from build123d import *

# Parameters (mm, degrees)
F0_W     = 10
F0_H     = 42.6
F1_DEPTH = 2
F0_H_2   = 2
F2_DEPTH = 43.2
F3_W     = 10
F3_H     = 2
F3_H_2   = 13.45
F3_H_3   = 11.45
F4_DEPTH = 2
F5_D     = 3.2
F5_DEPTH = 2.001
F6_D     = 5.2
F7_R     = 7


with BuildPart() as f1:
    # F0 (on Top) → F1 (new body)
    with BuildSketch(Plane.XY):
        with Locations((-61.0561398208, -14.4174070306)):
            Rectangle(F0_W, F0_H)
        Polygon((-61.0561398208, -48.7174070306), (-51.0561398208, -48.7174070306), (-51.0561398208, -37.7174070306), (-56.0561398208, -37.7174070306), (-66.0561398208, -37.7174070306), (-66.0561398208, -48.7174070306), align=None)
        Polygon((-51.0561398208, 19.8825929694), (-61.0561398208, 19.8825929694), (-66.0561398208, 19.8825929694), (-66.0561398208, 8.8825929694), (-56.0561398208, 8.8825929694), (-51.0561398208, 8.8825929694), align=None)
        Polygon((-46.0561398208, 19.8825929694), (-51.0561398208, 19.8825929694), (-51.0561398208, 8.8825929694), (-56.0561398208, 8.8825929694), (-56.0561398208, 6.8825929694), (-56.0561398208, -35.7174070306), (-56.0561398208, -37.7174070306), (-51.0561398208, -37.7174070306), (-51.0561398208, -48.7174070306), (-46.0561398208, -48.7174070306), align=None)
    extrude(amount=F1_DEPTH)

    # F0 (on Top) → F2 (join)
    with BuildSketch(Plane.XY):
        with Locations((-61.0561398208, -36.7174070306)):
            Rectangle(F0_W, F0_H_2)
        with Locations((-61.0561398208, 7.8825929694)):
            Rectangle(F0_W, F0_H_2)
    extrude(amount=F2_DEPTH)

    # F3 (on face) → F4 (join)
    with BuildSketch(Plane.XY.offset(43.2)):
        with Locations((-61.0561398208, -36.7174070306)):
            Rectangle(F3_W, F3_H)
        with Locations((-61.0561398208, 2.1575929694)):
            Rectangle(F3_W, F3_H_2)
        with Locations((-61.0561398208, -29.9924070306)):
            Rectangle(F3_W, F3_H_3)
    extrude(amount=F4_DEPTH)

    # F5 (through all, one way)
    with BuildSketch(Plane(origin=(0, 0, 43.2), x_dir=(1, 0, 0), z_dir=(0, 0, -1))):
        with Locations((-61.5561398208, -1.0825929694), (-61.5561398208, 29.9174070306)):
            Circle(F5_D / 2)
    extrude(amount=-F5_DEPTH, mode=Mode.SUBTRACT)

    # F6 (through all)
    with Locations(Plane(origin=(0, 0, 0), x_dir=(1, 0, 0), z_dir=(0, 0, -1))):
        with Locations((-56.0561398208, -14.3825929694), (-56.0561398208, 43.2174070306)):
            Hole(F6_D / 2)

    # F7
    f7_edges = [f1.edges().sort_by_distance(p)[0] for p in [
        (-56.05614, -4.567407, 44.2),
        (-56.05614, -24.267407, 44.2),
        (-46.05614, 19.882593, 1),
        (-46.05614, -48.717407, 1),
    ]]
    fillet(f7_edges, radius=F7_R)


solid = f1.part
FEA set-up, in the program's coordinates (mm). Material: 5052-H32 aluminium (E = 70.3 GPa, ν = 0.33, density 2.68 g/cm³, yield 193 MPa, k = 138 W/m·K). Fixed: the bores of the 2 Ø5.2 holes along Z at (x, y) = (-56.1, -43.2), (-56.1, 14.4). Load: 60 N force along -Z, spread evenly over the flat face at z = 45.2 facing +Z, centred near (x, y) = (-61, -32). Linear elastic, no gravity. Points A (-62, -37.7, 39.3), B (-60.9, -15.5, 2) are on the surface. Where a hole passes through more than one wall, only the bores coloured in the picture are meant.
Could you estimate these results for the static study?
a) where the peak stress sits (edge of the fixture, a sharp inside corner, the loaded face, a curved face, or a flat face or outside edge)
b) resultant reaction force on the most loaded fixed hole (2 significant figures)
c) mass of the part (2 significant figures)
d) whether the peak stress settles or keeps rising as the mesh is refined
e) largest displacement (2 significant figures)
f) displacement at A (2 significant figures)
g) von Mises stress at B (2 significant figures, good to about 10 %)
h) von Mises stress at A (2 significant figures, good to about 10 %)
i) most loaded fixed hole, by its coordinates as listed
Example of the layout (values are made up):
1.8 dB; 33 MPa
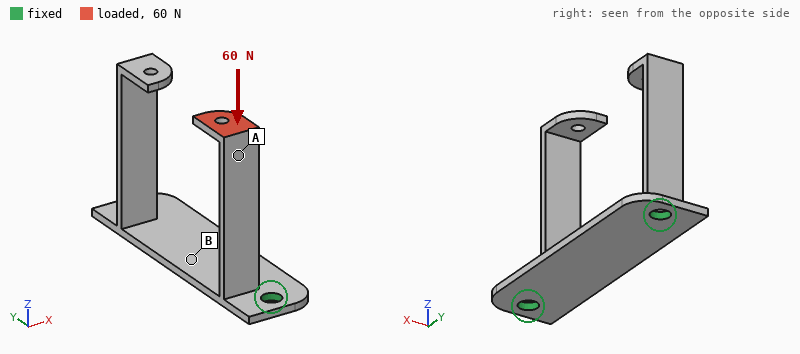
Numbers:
edge of the fixture; 55 N; 13 g; keeps rising; 0.85 mm; 0.56 mm; 5.5 MPa; 40 MPa; (-56.1, -43.2)
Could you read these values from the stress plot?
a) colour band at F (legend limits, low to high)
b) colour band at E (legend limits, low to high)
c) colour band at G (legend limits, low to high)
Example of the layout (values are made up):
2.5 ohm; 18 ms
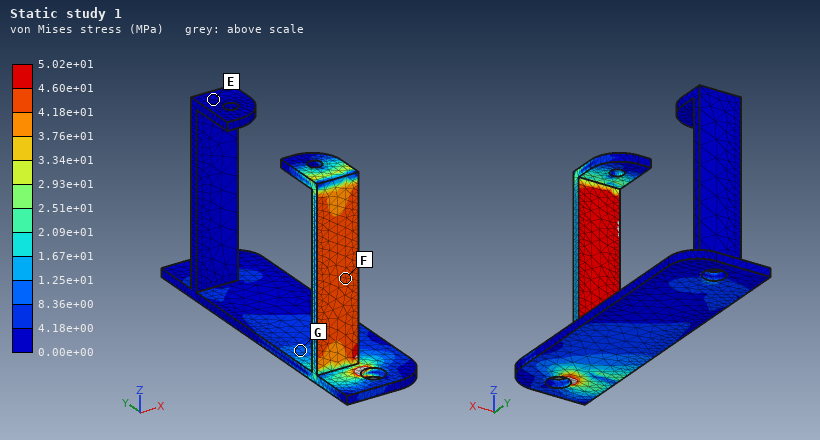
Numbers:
4.18e+01 to 4.60e+01 MPa; 0.00e+00 to 4.18e+00 MPa; 8.36e+00 to 1.25e+01 MPa
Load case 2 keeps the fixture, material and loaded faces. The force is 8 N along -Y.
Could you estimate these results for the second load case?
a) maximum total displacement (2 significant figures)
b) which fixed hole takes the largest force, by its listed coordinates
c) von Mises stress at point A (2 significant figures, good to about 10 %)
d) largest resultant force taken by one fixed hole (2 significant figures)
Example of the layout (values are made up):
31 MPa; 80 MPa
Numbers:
0.59 mm; (-56.1, -43.2); 7.0 MPa; 8.3 N
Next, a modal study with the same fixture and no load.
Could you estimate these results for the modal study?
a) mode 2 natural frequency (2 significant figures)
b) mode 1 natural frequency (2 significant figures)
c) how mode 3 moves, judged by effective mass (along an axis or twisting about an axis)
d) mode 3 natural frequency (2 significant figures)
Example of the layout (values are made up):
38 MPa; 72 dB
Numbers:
590 Hz; 570 Hz; along X; 1400 Hz
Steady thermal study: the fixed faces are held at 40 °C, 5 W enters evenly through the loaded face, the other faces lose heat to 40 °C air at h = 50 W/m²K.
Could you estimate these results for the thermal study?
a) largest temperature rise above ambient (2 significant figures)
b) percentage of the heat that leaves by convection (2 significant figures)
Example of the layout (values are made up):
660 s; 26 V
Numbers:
66 K; 45 %
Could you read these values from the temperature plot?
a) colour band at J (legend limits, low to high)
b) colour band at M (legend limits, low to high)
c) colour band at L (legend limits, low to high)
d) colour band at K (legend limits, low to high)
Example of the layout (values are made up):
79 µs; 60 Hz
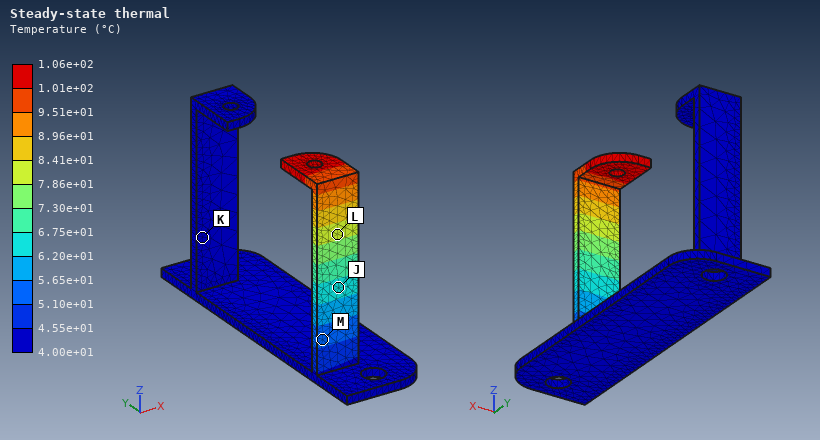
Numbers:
6.20e+01 to 6.75e+01 °C; 5.10e+01 to 5.65e+01 °C; 7.86e+01 to 8.41e+01 °C; 4.00e+01 to 4.55e+01 °C
